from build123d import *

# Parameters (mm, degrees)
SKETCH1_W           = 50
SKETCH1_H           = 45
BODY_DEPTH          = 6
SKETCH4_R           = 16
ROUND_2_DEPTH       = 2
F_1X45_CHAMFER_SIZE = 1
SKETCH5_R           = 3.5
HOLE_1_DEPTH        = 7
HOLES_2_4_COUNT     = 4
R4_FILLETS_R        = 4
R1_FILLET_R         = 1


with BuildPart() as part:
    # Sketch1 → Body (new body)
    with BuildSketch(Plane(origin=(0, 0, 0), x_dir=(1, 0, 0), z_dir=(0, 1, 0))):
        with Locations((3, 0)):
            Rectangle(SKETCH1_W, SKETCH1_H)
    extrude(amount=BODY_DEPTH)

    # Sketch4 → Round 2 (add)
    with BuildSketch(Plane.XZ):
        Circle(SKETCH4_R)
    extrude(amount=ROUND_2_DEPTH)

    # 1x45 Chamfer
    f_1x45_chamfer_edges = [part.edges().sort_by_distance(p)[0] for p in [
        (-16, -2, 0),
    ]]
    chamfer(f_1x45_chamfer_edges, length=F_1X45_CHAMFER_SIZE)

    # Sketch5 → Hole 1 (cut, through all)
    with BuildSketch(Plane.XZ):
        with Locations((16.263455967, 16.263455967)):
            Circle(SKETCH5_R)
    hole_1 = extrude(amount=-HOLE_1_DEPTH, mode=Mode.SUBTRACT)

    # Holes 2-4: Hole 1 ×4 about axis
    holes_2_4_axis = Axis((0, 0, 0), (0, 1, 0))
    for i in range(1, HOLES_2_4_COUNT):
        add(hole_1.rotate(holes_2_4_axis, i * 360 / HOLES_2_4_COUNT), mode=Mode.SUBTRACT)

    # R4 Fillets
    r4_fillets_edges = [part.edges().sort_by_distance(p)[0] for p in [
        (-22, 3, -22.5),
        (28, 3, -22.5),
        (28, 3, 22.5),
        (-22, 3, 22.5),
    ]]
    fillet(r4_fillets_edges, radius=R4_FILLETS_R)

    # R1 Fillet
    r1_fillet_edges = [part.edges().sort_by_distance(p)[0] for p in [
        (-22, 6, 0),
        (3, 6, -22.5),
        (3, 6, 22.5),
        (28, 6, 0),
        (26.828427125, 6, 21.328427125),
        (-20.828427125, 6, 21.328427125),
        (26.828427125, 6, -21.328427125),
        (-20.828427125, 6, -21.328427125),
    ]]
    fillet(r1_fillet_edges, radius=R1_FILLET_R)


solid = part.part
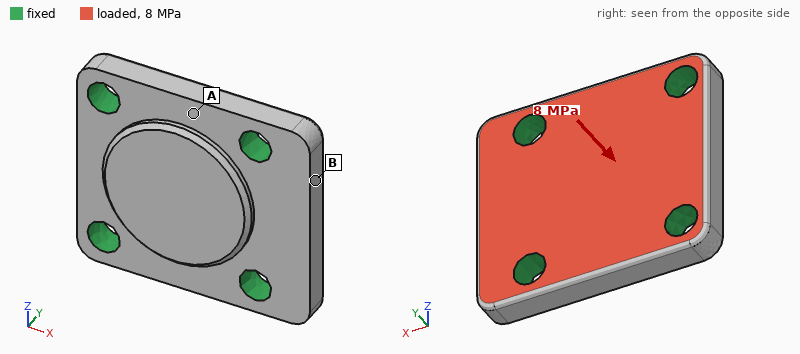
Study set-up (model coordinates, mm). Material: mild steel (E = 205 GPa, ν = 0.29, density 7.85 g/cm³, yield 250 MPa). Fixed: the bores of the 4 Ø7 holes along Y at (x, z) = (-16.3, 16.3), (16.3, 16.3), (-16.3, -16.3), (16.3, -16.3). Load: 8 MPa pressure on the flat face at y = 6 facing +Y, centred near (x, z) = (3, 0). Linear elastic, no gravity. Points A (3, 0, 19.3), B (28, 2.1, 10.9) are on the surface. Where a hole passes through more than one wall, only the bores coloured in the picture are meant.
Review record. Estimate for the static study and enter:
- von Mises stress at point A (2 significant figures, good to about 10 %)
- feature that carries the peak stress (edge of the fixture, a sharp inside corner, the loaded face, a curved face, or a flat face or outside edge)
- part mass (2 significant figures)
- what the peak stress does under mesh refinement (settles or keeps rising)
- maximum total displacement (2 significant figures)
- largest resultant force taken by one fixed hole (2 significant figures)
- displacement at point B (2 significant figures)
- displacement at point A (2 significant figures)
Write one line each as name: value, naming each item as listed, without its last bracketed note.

von Mises stress at point A: 33 MPa
feature that carries the peak stress: edge of the fixture
part mass: 110 g
what the peak stress does under mesh refinement: keeps rising
maximum total displacement: 8.5 µm
largest resultant force taken by one fixed hole: 4.4 kN
displacement at point B: 4.5 µm
displacement at point A: 4.3 µm
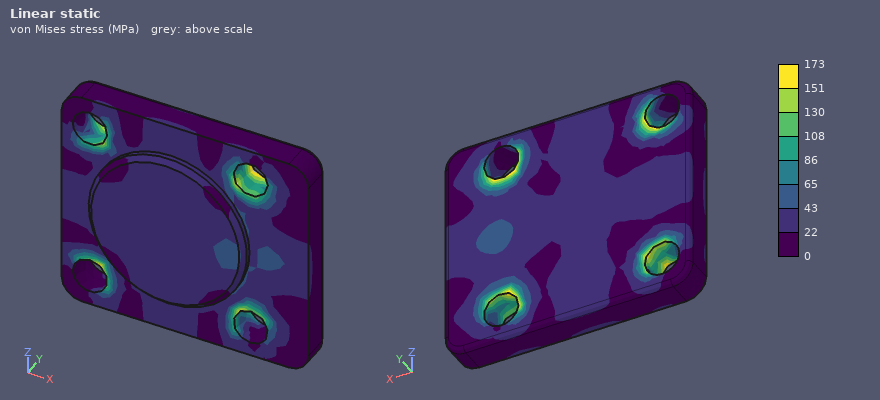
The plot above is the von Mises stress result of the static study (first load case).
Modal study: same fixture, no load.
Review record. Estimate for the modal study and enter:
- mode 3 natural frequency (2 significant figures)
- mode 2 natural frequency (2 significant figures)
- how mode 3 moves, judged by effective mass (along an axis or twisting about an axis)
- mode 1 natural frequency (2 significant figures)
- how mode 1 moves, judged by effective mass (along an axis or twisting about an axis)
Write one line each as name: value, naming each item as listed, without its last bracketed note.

mode 3 natural frequency: 34 kHz
mode 2 natural frequency: 27 kHz
how mode 3 moves, judged by effective mass: twisting about X
mode 1 natural frequency: 23 kHz
how mode 1 moves, judged by effective mass: along Y
